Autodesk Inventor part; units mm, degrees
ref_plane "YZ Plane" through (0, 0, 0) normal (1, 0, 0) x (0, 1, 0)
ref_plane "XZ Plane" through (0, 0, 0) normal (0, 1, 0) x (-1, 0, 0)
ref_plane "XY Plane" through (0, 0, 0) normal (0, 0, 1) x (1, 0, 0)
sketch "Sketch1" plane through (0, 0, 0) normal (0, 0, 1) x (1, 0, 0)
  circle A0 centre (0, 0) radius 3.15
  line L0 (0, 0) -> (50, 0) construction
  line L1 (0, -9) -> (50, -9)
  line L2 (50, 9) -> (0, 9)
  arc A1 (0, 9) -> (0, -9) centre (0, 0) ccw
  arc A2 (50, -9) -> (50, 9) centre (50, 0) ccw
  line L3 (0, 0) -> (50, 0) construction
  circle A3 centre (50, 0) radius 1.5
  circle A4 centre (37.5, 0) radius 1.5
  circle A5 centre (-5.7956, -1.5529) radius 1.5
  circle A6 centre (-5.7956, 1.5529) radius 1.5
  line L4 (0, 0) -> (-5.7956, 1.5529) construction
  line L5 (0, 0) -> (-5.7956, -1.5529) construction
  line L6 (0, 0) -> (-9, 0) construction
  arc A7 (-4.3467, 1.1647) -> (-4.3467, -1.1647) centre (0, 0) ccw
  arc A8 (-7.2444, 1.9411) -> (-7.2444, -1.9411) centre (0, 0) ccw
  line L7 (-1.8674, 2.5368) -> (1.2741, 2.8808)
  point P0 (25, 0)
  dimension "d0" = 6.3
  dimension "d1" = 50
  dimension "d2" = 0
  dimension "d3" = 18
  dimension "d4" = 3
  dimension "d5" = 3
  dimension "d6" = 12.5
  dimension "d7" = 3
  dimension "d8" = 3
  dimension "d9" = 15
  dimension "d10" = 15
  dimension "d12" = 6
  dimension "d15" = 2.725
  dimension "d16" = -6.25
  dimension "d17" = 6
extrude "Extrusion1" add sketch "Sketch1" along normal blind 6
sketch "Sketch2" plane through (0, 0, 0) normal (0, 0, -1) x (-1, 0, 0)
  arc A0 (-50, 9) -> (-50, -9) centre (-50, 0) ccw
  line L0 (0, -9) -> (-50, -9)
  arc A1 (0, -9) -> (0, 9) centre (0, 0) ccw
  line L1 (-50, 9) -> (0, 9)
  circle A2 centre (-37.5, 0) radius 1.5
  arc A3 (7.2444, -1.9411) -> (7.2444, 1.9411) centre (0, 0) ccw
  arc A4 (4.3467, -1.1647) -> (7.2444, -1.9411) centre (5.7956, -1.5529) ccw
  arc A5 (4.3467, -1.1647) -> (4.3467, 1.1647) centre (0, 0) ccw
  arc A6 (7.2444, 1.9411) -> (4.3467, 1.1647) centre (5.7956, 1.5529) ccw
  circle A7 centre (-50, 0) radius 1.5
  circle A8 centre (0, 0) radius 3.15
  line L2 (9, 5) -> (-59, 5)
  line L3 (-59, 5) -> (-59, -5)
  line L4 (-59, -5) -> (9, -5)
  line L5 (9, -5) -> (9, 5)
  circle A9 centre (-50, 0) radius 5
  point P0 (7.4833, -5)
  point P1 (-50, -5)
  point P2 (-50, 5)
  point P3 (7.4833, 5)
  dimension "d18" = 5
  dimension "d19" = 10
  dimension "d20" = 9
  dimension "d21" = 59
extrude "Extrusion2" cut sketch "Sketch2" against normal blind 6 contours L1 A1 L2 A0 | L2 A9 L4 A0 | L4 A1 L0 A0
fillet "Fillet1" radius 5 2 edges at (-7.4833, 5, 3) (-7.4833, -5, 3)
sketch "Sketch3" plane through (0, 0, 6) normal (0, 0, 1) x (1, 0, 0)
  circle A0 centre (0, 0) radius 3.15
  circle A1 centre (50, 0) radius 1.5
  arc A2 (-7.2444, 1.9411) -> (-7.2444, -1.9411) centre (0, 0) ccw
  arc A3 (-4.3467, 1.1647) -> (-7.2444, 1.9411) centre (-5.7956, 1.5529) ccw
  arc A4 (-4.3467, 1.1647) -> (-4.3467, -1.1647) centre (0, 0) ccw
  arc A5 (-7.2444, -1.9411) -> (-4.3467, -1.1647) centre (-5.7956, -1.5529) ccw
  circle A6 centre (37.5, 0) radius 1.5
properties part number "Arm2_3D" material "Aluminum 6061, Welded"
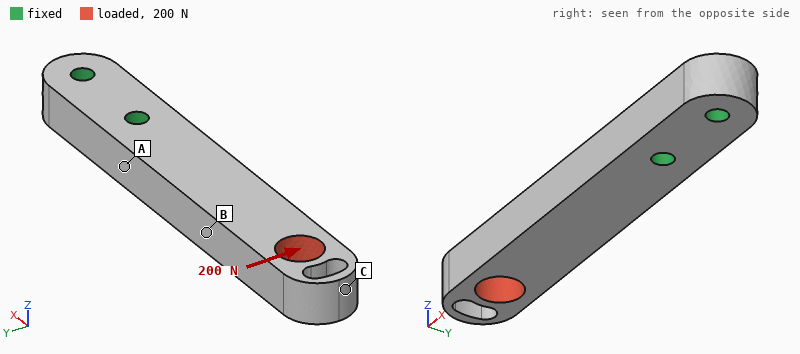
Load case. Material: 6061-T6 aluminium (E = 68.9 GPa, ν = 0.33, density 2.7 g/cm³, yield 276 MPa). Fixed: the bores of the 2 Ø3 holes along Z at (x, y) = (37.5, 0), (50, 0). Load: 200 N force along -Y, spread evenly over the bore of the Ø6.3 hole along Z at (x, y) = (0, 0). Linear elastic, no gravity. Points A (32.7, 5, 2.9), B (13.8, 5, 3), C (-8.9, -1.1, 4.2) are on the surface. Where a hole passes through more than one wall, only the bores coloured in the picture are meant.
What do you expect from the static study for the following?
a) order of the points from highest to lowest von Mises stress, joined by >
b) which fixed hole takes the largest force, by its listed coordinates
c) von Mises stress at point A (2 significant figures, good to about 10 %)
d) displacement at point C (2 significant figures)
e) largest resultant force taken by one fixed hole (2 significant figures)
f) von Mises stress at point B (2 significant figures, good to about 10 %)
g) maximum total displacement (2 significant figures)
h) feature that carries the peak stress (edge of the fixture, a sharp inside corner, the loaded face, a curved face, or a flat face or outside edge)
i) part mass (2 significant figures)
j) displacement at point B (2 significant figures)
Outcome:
A > B > C
(37.5, 0)
66 MPa
0.18 mm
510 N
28 MPa
0.18 mm
edge of the fixture
9.0 g
0.071 mm
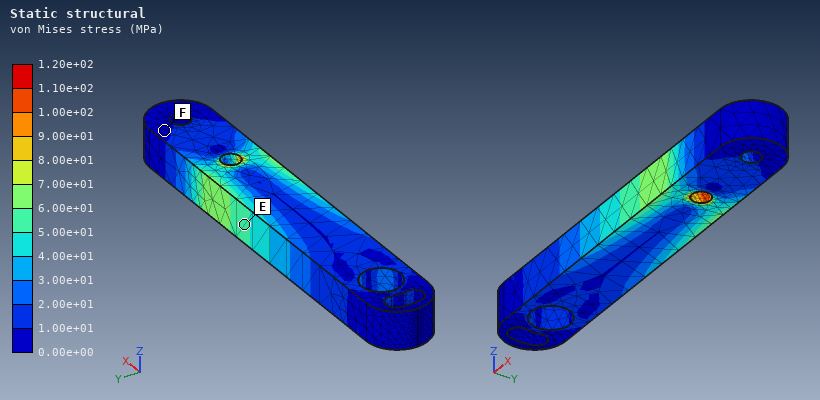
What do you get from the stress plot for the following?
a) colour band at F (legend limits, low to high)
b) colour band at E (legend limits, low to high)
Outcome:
0.00e+00 to 1.00e+01 MPa
5.00e+01 to 6.00e+01 MPa
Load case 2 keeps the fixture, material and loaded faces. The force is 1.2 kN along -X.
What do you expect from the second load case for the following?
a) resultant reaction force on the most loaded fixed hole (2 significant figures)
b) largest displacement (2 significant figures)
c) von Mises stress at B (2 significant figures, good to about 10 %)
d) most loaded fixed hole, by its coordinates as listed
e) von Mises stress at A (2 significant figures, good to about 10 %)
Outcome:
1.1 kN
18 µm
20 MPa
(37.5, 0)
16 MPa
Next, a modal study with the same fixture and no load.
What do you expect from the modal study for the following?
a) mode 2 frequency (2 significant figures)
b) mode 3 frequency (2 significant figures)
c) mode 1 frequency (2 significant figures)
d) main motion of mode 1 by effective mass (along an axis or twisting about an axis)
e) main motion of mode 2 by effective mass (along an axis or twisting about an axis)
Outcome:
4000 Hz
14 kHz
2800 Hz
along Z
along Y
